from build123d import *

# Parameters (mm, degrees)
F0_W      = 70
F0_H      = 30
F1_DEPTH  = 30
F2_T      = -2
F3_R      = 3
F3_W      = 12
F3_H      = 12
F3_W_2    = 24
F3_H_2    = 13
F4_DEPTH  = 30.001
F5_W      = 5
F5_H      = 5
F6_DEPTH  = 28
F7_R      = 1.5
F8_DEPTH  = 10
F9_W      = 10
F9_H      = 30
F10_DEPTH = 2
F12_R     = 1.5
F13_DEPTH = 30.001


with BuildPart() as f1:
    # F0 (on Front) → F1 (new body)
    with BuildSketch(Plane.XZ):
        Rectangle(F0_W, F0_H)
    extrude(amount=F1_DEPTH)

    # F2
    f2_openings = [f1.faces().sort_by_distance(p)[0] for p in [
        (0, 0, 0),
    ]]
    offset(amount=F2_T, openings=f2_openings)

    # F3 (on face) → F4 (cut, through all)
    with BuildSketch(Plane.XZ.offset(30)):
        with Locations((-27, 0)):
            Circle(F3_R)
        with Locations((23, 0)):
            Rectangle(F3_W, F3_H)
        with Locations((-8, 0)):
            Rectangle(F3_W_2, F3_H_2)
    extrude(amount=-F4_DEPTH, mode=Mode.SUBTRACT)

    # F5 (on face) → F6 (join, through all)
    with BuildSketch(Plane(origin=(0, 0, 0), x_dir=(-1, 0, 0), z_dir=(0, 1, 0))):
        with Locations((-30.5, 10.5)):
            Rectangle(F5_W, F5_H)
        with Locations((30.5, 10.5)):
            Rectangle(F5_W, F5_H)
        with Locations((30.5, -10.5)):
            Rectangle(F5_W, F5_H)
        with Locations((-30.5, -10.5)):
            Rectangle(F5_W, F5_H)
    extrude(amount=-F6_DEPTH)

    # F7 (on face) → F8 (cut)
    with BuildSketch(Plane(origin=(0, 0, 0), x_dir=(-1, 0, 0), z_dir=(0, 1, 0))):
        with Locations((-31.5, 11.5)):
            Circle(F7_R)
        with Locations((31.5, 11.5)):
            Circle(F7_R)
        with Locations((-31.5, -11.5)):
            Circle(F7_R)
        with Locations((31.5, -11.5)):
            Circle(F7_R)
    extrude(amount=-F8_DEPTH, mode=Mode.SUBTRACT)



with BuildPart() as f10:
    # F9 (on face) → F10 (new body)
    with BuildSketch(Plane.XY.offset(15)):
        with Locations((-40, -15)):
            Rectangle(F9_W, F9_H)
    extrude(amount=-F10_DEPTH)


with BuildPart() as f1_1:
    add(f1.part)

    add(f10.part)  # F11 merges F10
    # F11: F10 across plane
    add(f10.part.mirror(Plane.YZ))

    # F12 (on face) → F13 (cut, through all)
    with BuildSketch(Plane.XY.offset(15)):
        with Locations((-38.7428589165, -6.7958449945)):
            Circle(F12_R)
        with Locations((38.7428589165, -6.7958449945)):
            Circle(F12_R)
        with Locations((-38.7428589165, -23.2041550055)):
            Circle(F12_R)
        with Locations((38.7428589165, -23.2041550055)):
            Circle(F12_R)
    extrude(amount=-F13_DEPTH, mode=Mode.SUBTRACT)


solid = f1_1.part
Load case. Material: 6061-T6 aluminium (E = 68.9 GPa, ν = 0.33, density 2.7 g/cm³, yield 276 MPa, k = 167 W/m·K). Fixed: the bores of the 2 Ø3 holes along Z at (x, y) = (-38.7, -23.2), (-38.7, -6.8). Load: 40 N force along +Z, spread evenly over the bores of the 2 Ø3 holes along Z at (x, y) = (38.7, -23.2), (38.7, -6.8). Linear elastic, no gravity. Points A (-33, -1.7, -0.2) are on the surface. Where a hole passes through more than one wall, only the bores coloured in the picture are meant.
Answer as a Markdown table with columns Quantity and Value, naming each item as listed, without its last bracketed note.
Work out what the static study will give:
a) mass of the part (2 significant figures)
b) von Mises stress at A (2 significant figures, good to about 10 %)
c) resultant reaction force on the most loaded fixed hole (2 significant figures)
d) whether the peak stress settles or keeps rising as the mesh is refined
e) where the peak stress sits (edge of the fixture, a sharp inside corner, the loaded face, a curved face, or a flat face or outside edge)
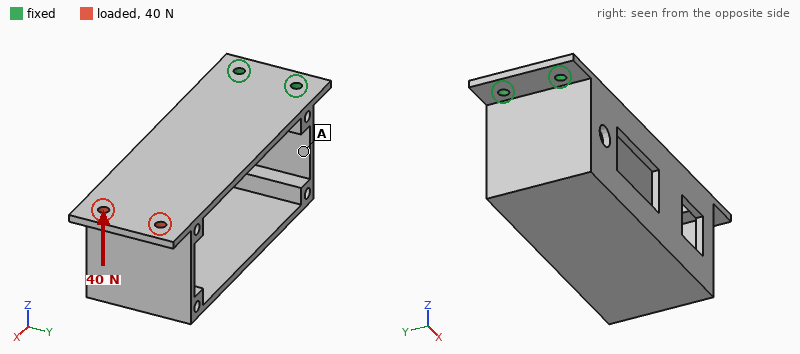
| Quantity | Value |
|---|---|
| mass of the part | 48 g |
| von Mises stress at A | 14 MPa |
| resultant reaction force on the most loaded fixed hole | 21 N |
| whether the peak stress settles or keeps rising as the mesh is refined | keeps rising |
| where the peak stress sits | edge of the fixture |
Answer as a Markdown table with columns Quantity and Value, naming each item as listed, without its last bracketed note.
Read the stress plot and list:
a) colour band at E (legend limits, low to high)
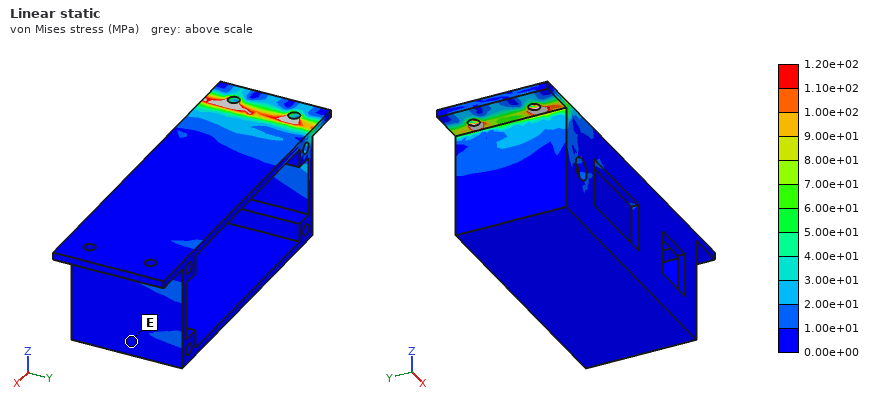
| Quantity | Value |
|---|---|
| colour band at E | 0.00e+00 to 1.00e+01 MPa |
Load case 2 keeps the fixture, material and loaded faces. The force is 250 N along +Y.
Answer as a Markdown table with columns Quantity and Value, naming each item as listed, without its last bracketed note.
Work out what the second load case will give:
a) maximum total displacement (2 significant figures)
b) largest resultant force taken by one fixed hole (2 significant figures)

| Quantity | Value |
|---|---|
| maximum total displacement | 0.16 mm |
| largest resultant force taken by one fixed hole | 1.1 kN |
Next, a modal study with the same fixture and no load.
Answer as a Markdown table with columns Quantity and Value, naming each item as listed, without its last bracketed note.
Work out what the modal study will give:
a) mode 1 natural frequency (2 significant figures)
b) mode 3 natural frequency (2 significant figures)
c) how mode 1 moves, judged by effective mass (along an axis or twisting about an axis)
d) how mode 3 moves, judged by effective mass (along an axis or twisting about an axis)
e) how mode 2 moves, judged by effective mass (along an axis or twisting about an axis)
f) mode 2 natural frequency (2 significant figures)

| Quantity | Value |
|---|---|
| mode 1 natural frequency | 240 Hz |
| mode 3 natural frequency | 2200 Hz |
| how mode 1 moves, judged by effective mass | along Z |
| how mode 3 moves, judged by effective mass | along Y |
| how mode 2 moves, judged by effective mass | along Y |
| mode 2 natural frequency | 950 Hz |
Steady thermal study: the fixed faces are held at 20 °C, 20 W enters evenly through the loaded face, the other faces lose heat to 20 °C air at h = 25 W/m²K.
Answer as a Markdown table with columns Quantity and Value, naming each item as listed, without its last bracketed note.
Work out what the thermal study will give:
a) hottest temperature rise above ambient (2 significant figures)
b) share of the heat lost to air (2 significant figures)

| Quantity | Value |
|---|---|
| hottest temperature rise above ambient | 64 K |
| share of the heat lost to air | 50 % |
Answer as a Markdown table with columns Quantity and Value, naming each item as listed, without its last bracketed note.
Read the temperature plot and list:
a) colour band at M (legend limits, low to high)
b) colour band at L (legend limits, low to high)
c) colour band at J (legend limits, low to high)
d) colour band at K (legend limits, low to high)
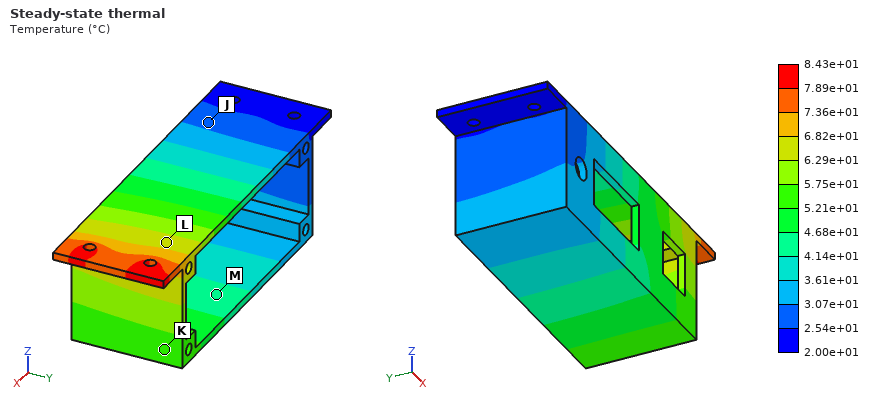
| Quantity | Value |
|---|---|
| colour band at M | 4.14e+01 to 4.68e+01 °C |
| colour band at L | 6.29e+01 to 6.82e+01 °C |
| colour band at J | 2.54e+01 to 3.07e+01 °C |
| colour band at K | 5.21e+01 to 5.75e+01 °C |
